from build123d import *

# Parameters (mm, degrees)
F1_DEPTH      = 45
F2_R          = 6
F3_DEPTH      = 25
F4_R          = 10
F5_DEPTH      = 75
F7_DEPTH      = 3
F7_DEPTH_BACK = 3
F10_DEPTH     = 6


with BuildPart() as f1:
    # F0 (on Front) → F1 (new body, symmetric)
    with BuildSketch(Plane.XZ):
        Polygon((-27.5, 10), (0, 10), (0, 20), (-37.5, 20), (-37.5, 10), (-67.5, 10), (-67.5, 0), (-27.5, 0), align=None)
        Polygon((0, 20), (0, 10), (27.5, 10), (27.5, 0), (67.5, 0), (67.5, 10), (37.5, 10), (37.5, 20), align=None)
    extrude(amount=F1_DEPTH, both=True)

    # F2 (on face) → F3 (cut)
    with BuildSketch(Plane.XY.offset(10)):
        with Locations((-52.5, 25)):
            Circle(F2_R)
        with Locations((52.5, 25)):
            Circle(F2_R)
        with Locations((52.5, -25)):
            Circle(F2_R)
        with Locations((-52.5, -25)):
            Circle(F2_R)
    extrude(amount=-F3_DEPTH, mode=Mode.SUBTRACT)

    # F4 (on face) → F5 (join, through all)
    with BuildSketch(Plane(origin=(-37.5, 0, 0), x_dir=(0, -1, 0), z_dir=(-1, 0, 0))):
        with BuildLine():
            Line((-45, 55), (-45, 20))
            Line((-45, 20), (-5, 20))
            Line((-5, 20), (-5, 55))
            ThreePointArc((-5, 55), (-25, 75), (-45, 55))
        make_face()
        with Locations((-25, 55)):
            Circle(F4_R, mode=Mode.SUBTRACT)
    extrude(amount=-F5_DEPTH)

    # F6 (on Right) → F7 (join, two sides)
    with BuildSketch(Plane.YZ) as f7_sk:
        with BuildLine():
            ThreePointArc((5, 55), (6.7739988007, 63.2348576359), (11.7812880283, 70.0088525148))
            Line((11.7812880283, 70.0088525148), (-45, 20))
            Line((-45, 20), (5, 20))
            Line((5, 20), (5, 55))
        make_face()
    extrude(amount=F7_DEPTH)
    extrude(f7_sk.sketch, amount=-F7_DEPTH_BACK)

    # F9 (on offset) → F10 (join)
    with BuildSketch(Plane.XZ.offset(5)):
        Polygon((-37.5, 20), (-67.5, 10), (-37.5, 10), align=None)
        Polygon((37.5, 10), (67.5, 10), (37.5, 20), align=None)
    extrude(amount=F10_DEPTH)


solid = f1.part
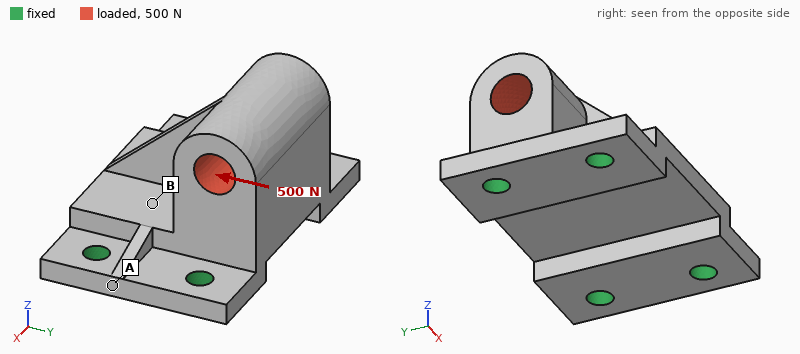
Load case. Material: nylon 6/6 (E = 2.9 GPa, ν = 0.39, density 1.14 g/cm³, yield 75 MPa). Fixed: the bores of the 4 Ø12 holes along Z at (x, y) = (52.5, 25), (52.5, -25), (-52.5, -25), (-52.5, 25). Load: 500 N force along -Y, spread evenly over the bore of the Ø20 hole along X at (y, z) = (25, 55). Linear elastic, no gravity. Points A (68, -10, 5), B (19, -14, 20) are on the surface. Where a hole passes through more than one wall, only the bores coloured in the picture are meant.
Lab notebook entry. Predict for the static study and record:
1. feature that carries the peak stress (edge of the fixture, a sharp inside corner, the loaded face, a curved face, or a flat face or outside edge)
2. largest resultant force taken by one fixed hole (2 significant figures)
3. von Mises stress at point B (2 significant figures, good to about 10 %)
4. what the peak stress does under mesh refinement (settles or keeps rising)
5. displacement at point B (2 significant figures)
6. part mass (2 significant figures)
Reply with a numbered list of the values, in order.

1. edge of the fixture
2. 410 N
3. 1.2 MPa
4. keeps rising
5. 0.040 mm
6. 310 g
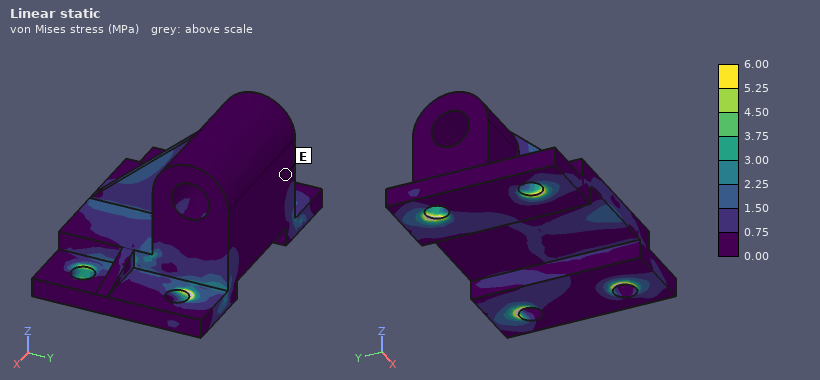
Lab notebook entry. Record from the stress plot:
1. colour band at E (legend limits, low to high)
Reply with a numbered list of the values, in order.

1. 0.00 to 0.75 MPa
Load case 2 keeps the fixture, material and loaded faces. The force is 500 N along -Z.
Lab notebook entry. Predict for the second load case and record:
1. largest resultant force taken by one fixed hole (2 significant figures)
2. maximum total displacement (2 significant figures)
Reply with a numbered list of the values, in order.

1. 290 N
2. 48 µm
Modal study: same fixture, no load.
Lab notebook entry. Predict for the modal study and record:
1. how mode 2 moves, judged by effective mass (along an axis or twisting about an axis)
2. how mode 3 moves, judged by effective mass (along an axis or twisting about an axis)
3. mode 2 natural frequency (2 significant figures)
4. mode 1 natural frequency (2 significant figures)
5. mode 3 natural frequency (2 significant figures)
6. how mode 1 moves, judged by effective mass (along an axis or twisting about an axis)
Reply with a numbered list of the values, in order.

1. along X
2. along Z
3. 1600 Hz
4. 910 Hz
5. 1600 Hz
6. along Y
